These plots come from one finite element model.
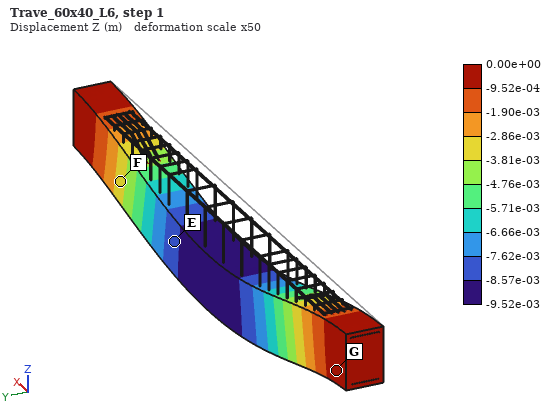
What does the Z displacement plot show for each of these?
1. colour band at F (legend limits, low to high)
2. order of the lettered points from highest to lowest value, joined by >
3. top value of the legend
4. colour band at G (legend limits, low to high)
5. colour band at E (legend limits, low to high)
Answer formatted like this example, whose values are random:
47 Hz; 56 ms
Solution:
-3.81e-03 to -2.86e-03 m; G > F > E; 0.00e+00 m; -9.52e-04 to 0.00e+00 m; -8.57e-03 to -7.62e-03 m
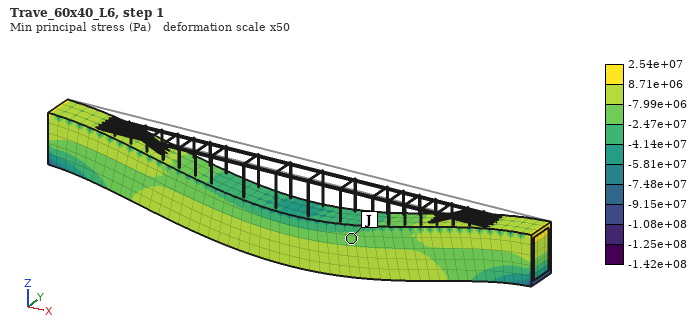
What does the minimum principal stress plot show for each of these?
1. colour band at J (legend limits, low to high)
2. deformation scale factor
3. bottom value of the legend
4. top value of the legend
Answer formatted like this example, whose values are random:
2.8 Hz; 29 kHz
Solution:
-2.47e+07 to -7.99e+06 Pa; 50; -1.42e+08 Pa; 2.54e+07 Pa
